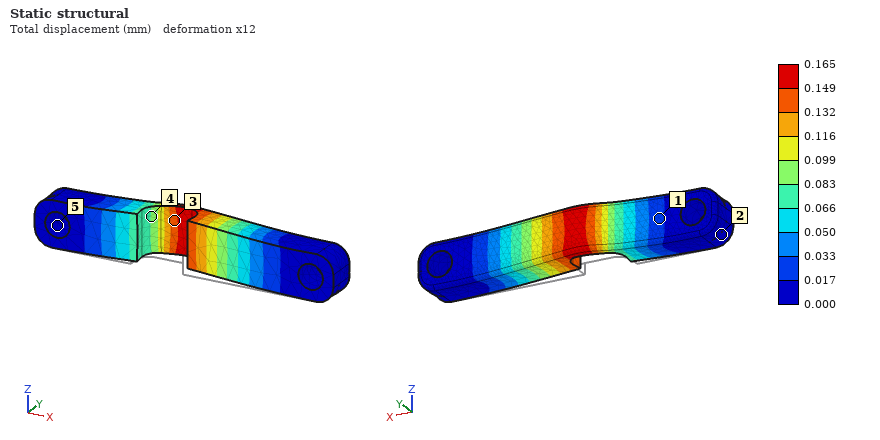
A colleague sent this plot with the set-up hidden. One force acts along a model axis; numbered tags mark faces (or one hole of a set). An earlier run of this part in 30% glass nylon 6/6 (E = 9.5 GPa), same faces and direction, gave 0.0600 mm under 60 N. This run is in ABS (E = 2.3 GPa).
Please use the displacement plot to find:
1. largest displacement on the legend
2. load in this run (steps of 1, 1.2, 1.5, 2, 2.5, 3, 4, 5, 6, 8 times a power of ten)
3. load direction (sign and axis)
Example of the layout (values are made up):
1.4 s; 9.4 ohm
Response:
0.165 mm; 40 N; +Y
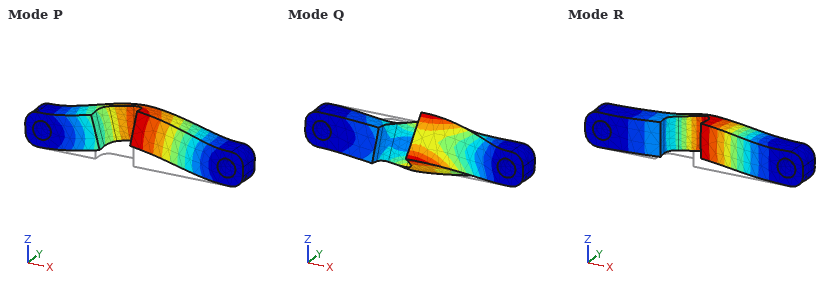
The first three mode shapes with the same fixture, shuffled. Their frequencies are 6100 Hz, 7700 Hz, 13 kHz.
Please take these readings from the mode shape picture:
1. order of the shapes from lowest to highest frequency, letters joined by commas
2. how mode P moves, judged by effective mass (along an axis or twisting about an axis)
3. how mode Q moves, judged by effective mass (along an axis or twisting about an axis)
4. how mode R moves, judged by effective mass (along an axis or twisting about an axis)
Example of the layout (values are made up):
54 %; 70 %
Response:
R, P, Q; along Z; twisting about X; along Y
